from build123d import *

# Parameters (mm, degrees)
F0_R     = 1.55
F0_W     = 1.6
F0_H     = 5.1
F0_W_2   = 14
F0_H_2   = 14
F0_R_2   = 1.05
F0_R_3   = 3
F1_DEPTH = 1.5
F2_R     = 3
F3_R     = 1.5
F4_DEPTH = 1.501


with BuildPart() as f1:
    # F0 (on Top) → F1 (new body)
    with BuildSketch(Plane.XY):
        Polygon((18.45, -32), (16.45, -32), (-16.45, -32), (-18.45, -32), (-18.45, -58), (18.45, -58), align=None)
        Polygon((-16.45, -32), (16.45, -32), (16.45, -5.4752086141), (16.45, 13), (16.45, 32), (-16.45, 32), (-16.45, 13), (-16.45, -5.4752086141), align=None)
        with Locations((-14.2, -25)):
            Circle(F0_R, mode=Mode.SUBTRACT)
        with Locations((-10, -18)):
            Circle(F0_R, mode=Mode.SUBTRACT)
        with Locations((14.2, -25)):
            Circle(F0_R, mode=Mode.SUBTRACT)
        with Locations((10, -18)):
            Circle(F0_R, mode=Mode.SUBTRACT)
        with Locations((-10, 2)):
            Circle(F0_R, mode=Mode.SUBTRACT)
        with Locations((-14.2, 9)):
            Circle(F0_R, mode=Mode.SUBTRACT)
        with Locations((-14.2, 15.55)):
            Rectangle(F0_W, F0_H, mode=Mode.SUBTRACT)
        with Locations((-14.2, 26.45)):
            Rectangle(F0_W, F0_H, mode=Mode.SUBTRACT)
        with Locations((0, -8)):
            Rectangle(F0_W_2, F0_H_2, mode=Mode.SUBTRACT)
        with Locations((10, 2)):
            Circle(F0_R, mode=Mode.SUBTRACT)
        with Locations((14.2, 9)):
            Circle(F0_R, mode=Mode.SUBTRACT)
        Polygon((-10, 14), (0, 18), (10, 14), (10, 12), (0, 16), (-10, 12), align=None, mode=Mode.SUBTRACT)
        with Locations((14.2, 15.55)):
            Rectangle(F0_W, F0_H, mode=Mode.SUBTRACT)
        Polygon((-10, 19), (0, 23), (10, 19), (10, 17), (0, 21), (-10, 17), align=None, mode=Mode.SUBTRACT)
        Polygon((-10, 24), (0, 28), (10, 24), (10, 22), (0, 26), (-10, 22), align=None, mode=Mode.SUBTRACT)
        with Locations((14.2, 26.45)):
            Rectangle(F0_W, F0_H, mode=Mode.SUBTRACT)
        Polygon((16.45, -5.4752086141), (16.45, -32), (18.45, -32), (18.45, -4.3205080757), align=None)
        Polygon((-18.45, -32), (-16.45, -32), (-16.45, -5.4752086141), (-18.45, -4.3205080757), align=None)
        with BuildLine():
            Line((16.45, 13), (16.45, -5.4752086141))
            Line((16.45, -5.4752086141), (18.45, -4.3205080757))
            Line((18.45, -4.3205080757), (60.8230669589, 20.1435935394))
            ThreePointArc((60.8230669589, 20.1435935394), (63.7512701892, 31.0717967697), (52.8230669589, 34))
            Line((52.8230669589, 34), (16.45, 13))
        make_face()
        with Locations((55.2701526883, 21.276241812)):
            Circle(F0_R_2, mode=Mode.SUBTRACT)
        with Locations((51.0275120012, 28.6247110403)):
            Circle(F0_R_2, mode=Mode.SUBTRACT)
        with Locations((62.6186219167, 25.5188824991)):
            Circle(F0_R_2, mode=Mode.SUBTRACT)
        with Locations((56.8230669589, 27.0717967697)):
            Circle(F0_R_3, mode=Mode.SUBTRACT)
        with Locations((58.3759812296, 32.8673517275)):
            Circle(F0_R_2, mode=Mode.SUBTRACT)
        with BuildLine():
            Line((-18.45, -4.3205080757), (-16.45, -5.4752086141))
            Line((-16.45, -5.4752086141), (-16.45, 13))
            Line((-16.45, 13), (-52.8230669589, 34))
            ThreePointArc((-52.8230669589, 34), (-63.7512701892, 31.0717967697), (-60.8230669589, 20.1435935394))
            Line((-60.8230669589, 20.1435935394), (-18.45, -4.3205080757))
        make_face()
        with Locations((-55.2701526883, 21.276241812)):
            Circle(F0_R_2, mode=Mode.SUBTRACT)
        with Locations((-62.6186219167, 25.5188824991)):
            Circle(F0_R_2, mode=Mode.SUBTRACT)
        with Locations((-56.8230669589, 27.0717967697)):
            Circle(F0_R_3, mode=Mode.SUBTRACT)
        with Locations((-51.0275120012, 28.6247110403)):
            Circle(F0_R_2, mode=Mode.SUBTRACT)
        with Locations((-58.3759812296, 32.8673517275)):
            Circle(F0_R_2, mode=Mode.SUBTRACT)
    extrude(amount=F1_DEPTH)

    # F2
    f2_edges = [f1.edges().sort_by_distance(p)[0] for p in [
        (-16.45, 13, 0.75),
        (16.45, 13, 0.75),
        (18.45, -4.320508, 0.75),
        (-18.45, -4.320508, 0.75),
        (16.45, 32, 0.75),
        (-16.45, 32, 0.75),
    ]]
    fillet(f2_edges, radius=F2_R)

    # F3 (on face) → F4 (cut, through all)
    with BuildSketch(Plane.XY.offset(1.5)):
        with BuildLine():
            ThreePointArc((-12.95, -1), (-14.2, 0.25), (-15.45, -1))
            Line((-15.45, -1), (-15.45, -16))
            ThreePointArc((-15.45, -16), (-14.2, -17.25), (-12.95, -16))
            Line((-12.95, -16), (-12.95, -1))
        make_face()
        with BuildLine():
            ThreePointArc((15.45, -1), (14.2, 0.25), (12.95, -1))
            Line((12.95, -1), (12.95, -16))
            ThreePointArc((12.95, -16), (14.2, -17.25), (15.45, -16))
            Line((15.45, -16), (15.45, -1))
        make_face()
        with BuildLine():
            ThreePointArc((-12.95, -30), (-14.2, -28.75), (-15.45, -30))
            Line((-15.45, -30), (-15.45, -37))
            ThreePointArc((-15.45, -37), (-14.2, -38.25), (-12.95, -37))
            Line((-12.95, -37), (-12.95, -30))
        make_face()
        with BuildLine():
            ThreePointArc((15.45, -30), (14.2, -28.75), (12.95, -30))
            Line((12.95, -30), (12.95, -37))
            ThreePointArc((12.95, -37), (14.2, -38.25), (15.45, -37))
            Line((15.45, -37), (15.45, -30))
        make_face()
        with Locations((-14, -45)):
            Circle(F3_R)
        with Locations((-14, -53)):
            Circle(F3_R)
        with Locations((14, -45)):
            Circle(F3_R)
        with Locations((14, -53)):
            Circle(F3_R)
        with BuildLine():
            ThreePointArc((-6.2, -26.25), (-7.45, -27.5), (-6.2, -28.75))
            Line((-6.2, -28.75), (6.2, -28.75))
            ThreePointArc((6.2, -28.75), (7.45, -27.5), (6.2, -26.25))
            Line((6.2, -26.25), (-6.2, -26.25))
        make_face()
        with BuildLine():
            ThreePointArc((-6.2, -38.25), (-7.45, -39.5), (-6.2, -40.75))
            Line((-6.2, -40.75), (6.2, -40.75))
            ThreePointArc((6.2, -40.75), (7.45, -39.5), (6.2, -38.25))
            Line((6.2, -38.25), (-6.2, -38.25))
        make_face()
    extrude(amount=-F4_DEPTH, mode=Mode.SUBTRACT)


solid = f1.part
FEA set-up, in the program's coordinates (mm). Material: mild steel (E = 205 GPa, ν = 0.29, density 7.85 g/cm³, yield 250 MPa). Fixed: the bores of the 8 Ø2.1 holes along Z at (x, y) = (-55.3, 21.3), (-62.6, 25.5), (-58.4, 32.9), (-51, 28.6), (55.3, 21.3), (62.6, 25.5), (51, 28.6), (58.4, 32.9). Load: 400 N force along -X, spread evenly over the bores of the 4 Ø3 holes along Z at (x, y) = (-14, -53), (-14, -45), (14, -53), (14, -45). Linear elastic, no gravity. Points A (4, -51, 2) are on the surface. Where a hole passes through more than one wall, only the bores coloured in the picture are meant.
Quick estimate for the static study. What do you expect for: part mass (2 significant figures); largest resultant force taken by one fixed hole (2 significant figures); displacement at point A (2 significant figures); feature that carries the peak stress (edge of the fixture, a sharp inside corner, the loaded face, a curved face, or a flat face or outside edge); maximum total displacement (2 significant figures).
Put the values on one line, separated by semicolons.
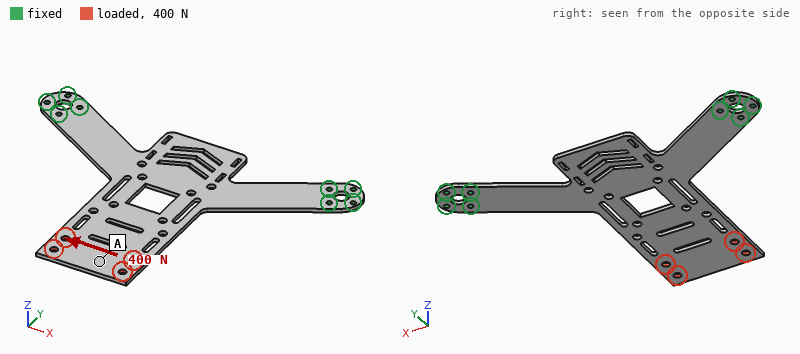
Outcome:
49 g; 460 N; 82 µm; a curved face; 94 µm
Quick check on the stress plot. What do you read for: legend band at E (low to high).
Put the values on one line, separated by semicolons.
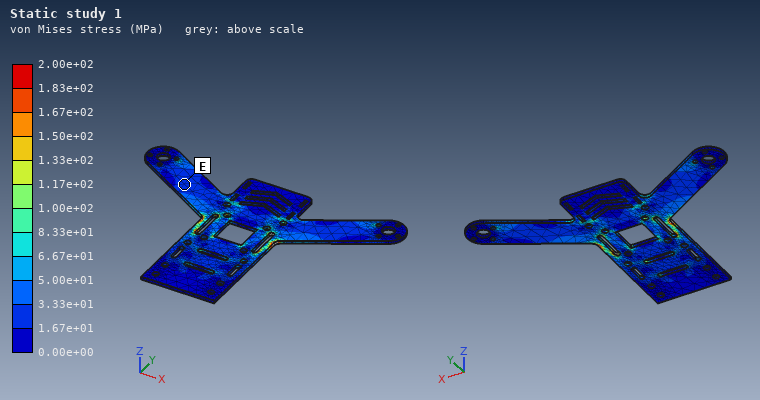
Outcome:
1.67e+01 to 3.33e+01 MPa
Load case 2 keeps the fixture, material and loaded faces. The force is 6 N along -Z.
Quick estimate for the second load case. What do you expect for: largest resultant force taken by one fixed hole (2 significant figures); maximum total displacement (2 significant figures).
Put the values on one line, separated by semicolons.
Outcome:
18 N; 0.79 mm
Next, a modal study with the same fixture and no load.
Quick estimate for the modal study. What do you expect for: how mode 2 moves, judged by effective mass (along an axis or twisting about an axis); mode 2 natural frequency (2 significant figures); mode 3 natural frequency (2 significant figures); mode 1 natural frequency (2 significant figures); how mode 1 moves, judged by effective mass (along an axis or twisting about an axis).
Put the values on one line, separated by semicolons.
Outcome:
along Z; 540 Hz; 810 Hz; 140 Hz; along Z
